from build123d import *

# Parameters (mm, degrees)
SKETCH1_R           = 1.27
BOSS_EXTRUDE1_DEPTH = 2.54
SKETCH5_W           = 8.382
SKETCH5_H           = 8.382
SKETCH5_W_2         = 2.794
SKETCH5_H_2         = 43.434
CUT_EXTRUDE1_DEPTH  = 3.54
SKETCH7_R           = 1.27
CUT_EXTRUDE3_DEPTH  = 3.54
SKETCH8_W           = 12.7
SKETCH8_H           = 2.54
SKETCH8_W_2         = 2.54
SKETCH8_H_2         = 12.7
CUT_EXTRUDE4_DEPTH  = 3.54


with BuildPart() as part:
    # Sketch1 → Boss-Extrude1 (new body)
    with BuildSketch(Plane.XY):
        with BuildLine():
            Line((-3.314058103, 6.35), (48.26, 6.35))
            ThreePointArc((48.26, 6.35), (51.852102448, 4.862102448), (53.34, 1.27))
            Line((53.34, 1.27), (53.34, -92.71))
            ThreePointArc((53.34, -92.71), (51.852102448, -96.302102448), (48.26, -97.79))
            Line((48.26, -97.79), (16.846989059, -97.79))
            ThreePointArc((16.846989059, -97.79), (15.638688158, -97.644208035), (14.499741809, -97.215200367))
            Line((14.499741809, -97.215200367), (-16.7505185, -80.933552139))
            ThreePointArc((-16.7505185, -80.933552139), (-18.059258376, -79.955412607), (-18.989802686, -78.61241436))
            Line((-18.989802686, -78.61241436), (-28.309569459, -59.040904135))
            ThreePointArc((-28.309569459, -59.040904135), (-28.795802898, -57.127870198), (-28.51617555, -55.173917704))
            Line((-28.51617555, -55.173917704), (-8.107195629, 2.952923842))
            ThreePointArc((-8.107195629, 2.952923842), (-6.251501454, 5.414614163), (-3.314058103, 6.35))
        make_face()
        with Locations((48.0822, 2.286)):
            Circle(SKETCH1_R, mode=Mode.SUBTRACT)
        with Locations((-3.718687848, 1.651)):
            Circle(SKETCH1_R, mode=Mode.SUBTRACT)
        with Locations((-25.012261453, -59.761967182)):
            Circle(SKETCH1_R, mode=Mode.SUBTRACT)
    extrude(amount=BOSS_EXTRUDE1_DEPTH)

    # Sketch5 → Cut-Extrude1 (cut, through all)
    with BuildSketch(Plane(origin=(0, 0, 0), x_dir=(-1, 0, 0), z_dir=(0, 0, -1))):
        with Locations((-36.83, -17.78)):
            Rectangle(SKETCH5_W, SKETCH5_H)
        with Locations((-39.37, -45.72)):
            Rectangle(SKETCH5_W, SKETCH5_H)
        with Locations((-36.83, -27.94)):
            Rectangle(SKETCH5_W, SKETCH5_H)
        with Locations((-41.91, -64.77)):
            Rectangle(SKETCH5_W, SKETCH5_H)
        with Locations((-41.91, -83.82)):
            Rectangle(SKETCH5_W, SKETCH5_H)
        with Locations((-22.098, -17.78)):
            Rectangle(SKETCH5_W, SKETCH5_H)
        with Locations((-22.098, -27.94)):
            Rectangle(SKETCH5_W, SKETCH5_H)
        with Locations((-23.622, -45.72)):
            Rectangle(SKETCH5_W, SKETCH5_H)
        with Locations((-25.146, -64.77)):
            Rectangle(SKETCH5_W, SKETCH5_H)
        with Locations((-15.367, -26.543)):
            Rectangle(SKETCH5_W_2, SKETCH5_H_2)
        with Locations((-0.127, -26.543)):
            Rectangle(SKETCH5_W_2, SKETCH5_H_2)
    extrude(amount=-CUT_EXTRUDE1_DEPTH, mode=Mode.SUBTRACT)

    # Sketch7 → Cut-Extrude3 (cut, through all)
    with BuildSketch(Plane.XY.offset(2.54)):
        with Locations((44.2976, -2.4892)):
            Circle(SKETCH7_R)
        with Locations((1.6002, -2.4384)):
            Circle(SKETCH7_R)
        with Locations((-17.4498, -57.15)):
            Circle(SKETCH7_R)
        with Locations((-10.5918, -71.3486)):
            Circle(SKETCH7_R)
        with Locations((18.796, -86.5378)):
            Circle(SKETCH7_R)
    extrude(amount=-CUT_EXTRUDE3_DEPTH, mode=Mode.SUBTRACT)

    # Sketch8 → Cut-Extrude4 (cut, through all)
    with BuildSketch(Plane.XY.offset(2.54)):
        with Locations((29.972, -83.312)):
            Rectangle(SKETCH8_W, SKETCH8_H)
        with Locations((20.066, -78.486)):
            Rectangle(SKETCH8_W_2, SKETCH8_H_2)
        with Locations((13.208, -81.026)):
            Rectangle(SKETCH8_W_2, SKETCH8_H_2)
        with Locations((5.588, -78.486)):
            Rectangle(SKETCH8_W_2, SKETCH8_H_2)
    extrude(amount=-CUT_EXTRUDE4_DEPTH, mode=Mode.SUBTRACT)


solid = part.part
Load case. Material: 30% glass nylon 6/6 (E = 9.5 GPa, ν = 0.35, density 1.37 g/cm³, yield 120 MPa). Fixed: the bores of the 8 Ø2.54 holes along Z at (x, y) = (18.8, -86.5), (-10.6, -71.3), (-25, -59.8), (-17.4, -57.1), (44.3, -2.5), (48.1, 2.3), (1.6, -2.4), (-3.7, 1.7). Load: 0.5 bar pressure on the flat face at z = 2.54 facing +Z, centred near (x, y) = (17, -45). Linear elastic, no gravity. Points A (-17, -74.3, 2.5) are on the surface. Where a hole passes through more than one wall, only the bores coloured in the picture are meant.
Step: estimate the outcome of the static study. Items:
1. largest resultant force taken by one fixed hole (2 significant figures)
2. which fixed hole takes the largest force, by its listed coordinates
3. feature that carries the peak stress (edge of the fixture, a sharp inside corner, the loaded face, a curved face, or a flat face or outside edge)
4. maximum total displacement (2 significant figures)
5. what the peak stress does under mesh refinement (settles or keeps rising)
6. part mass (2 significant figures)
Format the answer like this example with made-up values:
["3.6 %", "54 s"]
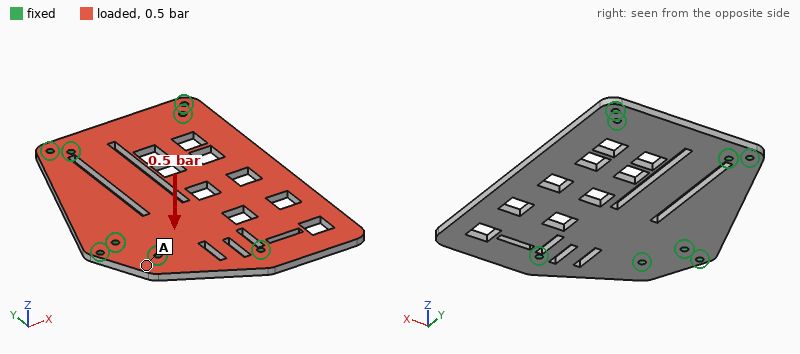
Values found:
["120 N", "(44.3, -2.5)", "edge of the fixture", "1.5 mm", "keeps rising", "22 g"]
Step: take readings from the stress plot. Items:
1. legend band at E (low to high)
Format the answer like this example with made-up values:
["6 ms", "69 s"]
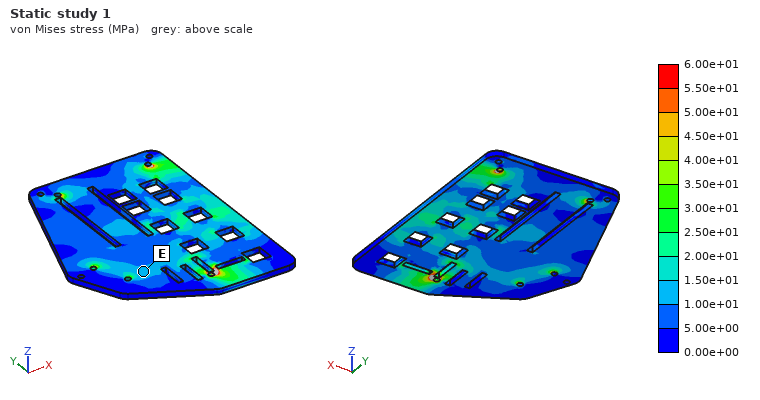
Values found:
["1.00e+01 to 1.50e+01 MPa"]
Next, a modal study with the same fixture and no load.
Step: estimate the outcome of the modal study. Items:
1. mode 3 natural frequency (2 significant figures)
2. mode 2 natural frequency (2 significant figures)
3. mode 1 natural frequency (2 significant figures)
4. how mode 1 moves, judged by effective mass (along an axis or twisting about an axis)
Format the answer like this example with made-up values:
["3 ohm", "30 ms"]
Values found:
["1600 Hz", "1100 Hz", "650 Hz", "along Z"]
